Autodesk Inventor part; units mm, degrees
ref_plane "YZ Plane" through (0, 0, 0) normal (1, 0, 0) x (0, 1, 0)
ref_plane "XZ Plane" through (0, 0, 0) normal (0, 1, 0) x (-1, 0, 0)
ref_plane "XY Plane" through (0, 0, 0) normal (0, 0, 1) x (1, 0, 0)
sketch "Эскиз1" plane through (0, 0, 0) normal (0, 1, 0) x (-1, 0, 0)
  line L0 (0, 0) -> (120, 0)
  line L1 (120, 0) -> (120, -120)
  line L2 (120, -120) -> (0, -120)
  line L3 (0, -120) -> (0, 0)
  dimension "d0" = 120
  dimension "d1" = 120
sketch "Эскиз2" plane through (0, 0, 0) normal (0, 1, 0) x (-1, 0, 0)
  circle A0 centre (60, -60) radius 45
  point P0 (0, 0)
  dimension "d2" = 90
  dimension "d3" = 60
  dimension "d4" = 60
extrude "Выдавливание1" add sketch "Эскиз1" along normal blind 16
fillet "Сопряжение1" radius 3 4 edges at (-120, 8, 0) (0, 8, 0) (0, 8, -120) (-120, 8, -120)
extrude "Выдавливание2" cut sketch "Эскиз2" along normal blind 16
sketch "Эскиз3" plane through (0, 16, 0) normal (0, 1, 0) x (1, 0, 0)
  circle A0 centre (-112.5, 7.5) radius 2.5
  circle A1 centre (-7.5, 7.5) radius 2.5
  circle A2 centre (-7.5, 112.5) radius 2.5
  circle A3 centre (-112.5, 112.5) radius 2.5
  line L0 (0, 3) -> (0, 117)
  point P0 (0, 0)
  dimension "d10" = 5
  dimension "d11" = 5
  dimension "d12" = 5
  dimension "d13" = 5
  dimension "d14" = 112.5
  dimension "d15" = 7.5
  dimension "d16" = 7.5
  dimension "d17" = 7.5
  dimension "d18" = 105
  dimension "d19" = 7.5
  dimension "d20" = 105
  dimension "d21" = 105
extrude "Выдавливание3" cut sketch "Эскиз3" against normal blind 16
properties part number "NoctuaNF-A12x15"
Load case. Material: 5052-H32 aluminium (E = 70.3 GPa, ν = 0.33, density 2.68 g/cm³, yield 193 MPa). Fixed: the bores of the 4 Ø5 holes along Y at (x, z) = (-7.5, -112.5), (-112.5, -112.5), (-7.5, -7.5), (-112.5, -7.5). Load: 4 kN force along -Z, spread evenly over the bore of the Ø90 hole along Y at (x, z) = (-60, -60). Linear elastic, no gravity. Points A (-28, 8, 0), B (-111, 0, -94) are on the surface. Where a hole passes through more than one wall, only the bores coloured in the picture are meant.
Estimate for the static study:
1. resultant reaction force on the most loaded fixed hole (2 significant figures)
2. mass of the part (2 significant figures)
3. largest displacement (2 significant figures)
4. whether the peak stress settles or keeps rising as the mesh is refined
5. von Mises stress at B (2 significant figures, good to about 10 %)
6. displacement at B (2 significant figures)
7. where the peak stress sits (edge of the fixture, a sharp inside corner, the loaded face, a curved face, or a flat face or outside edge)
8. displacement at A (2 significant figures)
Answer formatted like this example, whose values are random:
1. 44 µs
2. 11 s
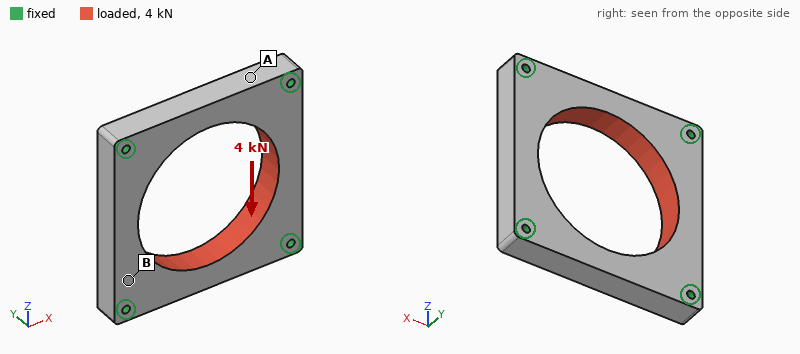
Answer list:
1. 1.0 kN
2. 340 g
3. 7.6 µm
4. keeps rising
5. 2.7 MPa
6. 2.0 µm
7. edge of the fixture
8. 3.5 µm
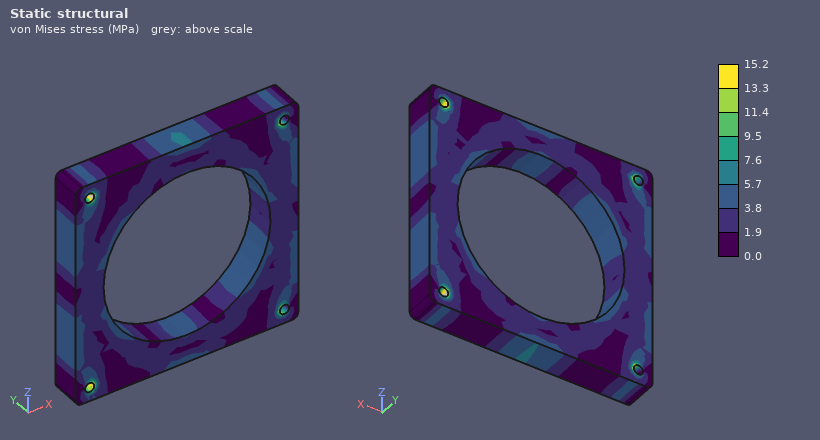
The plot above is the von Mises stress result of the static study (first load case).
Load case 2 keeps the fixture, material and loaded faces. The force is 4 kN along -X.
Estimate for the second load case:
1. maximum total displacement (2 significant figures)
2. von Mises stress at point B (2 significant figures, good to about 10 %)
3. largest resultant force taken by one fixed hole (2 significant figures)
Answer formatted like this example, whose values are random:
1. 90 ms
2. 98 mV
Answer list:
1. 7.6 µm
2. 1.6 MPa
3. 1.0 kN
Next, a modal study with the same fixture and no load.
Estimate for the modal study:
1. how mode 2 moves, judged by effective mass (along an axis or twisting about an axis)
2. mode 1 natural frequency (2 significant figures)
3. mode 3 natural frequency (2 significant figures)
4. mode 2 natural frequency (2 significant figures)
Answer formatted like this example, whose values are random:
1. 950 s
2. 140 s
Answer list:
1. along Y
2. 4700 Hz
3. 6800 Hz
4. 6200 Hz
